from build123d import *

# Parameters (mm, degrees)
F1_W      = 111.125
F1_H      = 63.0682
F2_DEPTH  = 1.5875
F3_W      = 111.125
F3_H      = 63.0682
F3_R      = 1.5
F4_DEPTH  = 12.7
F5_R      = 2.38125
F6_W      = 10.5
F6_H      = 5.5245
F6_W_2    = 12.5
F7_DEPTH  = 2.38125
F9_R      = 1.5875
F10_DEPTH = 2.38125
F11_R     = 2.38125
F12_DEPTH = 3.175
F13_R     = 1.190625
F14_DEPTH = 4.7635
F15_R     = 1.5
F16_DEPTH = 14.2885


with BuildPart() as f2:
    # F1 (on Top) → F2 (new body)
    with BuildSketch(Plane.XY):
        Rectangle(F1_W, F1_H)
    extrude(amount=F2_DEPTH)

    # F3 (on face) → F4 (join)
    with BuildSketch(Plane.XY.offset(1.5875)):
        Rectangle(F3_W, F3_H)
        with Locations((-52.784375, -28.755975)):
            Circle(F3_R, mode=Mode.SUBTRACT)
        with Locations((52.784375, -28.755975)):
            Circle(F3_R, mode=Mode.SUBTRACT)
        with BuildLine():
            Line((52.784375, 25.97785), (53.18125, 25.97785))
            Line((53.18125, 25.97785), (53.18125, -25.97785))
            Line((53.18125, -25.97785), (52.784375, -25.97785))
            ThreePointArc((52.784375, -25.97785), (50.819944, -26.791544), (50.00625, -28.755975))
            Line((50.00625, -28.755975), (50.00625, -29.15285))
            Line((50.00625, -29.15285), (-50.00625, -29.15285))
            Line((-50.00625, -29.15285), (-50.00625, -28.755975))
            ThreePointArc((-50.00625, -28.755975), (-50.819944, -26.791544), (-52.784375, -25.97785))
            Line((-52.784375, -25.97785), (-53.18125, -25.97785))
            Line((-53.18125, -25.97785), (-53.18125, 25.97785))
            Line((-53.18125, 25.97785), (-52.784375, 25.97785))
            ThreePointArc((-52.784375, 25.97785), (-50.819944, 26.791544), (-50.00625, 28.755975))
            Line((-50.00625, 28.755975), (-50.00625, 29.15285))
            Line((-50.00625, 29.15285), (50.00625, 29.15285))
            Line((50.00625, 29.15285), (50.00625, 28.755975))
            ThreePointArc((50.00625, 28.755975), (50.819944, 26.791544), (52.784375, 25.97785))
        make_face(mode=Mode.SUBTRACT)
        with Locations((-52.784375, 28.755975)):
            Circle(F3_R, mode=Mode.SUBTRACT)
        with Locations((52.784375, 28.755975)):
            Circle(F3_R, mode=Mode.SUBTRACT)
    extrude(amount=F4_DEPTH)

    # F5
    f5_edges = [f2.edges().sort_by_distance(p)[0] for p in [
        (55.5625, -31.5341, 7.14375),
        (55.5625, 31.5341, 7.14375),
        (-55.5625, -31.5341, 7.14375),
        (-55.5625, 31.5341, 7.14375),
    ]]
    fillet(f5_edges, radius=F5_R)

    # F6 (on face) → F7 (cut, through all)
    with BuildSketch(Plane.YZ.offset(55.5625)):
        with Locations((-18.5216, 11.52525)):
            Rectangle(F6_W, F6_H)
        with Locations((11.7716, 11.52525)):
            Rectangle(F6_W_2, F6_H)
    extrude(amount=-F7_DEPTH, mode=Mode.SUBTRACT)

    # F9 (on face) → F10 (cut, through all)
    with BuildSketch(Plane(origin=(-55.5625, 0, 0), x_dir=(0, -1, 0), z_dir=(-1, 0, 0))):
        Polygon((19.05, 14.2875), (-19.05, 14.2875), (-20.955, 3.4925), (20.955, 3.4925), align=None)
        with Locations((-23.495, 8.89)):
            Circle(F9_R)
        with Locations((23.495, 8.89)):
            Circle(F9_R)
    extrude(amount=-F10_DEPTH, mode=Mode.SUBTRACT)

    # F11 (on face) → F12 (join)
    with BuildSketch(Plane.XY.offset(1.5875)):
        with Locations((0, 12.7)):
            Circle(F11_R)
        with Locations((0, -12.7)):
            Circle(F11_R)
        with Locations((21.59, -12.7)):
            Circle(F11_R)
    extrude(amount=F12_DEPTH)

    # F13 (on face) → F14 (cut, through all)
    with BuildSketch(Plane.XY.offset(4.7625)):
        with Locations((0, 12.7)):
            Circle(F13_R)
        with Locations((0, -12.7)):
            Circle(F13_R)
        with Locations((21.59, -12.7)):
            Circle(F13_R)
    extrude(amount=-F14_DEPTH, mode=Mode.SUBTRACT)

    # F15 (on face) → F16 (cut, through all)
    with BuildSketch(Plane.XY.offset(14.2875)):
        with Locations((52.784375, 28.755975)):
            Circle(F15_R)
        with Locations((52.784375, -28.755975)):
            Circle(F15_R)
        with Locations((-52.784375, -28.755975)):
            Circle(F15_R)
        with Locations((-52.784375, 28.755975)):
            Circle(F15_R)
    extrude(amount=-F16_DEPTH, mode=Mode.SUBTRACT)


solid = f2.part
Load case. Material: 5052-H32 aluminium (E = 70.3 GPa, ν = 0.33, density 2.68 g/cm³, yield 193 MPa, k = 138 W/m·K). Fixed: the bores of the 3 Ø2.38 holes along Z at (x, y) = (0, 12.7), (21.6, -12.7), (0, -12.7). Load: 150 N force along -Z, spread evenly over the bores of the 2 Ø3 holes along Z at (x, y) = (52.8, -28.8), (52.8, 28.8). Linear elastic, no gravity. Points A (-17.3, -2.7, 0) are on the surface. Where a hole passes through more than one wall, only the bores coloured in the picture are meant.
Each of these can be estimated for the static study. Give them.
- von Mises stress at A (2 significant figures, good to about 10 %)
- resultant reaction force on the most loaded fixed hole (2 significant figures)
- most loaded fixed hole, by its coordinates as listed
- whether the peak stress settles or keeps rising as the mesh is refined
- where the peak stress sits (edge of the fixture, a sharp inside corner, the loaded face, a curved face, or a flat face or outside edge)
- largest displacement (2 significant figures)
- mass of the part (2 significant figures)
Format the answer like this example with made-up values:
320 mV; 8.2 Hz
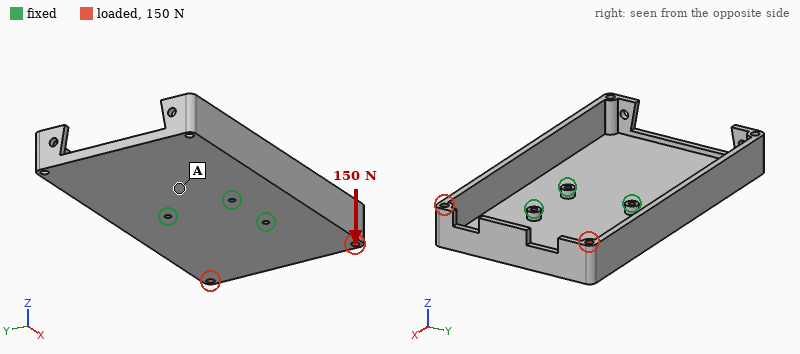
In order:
16 MPa; 240 N; (21.6, -12.7); keeps rising; edge of the fixture; 0.81 mm; 54 g
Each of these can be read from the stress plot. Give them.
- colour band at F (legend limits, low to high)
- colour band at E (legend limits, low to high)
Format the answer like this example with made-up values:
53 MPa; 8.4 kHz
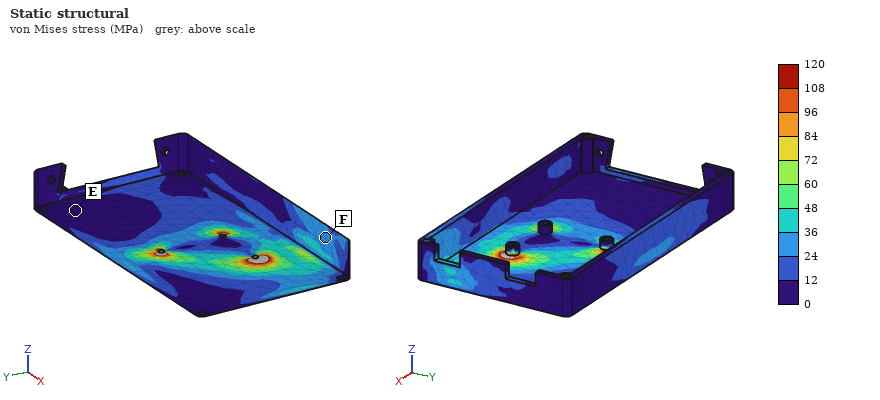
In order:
24 to 36 MPa; 0 to 12 MPa
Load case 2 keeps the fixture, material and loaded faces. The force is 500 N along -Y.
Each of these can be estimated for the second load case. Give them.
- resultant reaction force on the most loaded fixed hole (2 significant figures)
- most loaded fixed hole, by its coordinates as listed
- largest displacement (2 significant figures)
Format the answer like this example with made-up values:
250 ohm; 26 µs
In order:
720 N; (21.6, -12.7); 0.62 mm
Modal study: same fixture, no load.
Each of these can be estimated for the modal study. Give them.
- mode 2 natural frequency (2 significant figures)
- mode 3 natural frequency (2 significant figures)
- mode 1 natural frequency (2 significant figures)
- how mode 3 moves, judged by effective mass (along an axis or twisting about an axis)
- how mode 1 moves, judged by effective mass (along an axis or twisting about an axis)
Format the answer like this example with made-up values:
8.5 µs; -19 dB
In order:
790 Hz; 970 Hz; 520 Hz; along Z; twisting about Y
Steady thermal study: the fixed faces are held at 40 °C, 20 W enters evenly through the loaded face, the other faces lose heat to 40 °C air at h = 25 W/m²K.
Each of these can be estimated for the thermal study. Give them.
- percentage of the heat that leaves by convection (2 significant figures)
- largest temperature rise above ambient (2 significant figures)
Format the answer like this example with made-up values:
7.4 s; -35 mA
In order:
34 %; 44 K
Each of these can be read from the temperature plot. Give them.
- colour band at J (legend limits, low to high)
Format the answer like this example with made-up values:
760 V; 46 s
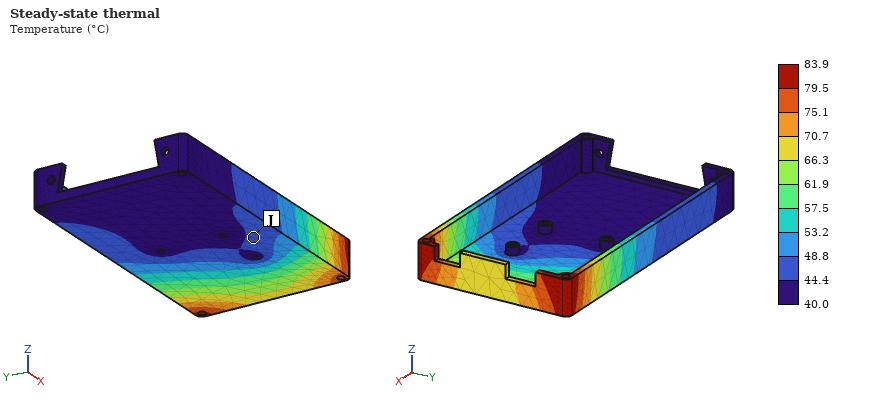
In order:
44.4 to 48.8 °C
